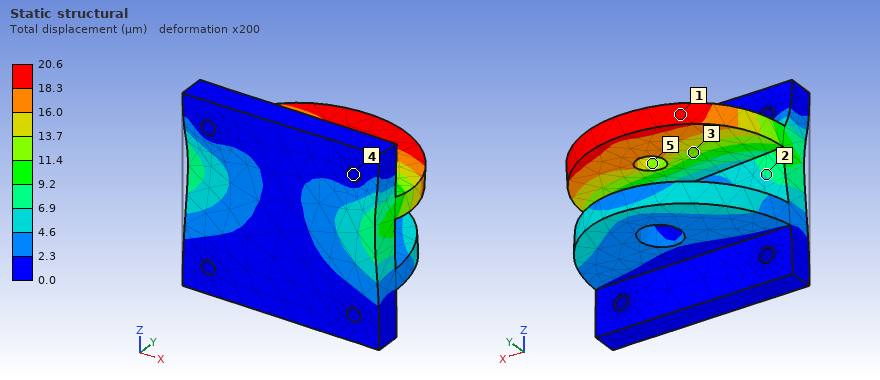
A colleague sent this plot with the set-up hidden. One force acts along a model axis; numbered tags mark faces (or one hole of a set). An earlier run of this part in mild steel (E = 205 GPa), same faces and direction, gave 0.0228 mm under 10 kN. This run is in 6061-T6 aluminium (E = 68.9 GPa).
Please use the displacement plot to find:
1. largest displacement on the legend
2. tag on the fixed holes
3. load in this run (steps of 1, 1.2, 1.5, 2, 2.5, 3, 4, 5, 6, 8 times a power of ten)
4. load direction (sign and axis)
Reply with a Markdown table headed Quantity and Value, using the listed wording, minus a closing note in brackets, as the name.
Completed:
| Quantity | Value |
|---|---|
| largest displacement on the legend | 20.6 µm |
| tag on the fixed holes | 4 |
| load in this run | 3 kN |
| load direction | +X |
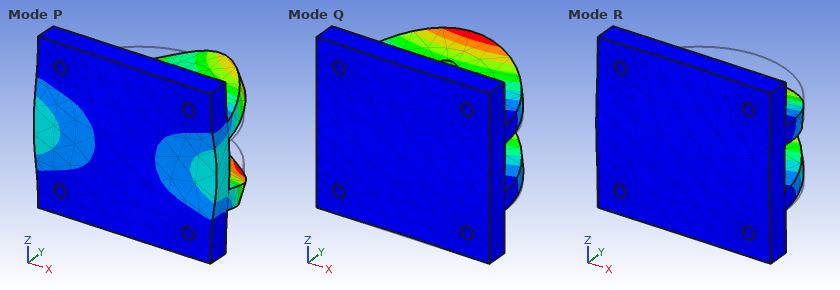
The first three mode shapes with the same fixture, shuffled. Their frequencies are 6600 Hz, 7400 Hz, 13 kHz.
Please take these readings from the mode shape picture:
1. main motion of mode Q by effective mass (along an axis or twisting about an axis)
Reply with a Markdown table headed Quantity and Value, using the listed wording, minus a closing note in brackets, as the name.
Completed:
| Quantity | Value |
|---|---|
| main motion of mode Q by effective mass | along Z |
